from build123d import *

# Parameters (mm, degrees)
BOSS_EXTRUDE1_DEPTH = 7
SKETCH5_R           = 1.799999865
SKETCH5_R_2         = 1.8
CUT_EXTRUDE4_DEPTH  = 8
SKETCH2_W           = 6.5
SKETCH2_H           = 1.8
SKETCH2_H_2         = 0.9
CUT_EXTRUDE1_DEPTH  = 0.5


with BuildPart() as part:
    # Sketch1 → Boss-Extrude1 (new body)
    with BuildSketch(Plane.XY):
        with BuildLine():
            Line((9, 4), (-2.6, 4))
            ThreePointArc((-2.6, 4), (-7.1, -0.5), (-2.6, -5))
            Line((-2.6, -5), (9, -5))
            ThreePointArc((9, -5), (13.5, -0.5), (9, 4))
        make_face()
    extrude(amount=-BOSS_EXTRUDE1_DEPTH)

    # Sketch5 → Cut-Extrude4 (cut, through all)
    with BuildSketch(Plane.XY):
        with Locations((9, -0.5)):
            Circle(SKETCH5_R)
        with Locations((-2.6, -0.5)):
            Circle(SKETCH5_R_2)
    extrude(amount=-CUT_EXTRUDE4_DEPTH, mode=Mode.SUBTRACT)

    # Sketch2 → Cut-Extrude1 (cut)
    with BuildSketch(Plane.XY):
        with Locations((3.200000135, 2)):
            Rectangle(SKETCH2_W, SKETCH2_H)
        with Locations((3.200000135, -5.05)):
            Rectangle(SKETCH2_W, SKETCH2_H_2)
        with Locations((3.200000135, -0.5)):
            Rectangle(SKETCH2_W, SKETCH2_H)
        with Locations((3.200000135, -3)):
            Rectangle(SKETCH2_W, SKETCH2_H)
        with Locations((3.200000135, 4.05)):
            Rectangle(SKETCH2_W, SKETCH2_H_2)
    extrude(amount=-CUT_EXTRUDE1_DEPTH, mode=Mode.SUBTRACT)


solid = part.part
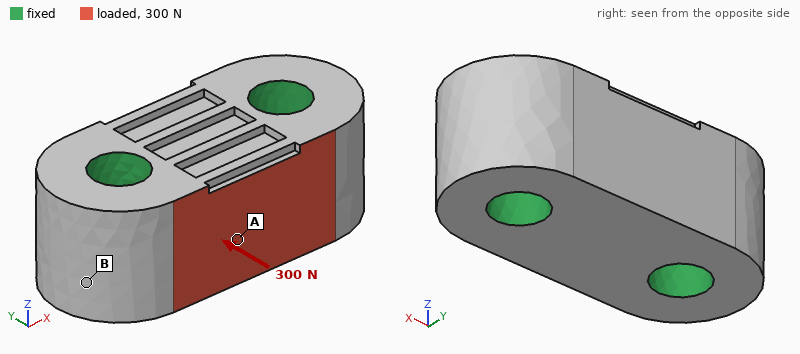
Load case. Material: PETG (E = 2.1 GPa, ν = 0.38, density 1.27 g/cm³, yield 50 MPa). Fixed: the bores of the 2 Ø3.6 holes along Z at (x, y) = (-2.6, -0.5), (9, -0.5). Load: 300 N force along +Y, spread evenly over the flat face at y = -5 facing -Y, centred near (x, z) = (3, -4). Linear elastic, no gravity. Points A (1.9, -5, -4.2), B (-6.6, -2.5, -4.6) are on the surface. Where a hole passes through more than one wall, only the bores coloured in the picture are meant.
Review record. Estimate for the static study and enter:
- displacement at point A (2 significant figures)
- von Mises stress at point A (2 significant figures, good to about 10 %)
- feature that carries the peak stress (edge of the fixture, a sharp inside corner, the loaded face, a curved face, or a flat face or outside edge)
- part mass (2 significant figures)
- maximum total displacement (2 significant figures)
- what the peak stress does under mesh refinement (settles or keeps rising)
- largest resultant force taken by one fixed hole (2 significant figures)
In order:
12 µm
3.7 MPa
edge of the fixture
1.3 g
15 µm
keeps rising
160 N
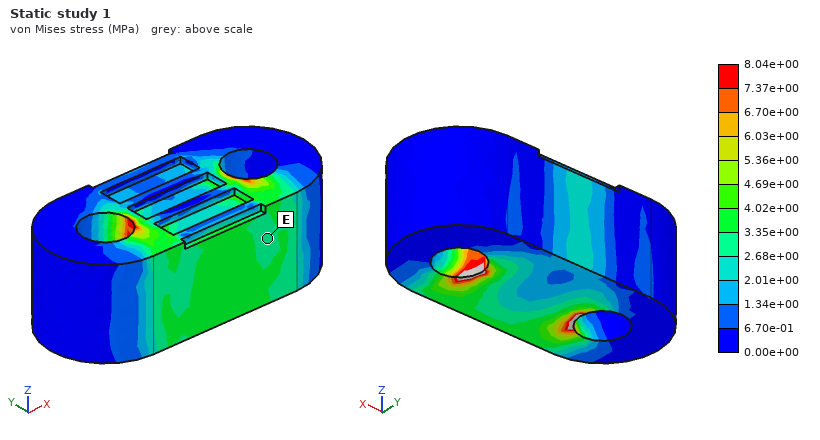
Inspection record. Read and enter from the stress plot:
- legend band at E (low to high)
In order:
2.68e+00 to 3.35e+00 MPa
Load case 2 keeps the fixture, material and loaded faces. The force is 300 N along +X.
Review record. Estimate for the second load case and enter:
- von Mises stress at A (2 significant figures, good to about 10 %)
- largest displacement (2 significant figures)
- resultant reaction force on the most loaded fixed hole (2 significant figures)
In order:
6.7 MPa
16 µm
170 N
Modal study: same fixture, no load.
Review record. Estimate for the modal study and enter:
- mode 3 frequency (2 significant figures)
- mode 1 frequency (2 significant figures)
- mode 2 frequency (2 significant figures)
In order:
34 kHz
33 kHz
33 kHz
